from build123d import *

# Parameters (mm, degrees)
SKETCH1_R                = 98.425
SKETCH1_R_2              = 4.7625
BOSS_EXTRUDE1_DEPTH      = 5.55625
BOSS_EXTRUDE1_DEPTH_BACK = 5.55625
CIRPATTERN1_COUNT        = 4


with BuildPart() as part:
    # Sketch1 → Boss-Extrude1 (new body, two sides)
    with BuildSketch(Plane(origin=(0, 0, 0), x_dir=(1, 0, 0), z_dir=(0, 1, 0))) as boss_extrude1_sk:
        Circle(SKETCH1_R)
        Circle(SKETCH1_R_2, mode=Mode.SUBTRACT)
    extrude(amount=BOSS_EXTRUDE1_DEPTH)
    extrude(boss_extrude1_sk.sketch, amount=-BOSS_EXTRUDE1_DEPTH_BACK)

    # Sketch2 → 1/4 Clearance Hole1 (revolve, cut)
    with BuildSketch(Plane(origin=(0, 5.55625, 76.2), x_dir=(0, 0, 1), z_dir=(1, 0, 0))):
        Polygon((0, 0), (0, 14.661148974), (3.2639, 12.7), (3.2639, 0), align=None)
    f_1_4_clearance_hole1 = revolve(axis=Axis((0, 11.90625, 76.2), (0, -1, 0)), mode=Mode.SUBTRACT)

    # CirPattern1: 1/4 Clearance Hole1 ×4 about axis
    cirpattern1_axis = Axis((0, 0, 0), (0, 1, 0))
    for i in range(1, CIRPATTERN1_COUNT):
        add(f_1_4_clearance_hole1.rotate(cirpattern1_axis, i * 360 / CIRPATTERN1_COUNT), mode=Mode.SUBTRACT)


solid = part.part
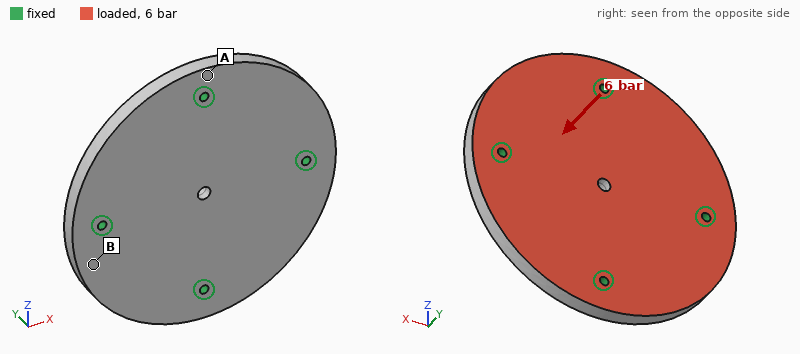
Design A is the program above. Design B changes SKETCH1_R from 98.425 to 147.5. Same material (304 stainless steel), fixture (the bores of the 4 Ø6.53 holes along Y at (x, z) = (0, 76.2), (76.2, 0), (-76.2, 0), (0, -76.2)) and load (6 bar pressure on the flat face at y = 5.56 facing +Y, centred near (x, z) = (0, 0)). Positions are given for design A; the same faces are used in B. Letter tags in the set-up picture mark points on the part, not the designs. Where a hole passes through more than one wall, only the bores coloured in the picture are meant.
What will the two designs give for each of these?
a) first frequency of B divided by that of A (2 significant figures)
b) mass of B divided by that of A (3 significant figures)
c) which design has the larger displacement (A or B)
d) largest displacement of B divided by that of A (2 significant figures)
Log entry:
0.35
2.25
B
8.3
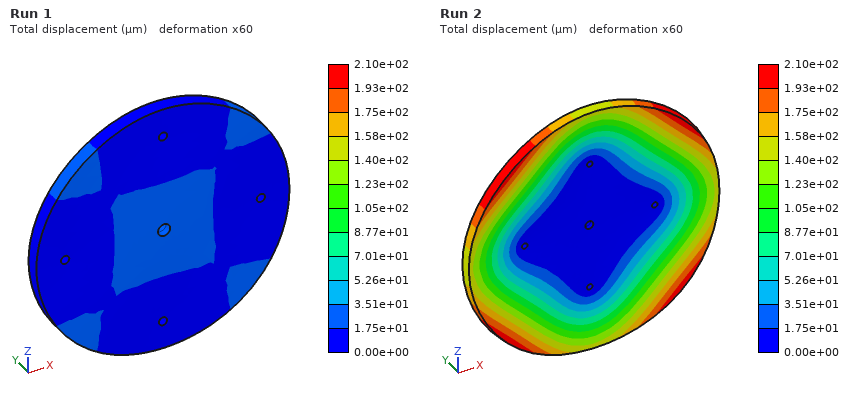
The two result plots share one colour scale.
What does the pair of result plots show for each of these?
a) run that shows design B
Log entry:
Run 2
